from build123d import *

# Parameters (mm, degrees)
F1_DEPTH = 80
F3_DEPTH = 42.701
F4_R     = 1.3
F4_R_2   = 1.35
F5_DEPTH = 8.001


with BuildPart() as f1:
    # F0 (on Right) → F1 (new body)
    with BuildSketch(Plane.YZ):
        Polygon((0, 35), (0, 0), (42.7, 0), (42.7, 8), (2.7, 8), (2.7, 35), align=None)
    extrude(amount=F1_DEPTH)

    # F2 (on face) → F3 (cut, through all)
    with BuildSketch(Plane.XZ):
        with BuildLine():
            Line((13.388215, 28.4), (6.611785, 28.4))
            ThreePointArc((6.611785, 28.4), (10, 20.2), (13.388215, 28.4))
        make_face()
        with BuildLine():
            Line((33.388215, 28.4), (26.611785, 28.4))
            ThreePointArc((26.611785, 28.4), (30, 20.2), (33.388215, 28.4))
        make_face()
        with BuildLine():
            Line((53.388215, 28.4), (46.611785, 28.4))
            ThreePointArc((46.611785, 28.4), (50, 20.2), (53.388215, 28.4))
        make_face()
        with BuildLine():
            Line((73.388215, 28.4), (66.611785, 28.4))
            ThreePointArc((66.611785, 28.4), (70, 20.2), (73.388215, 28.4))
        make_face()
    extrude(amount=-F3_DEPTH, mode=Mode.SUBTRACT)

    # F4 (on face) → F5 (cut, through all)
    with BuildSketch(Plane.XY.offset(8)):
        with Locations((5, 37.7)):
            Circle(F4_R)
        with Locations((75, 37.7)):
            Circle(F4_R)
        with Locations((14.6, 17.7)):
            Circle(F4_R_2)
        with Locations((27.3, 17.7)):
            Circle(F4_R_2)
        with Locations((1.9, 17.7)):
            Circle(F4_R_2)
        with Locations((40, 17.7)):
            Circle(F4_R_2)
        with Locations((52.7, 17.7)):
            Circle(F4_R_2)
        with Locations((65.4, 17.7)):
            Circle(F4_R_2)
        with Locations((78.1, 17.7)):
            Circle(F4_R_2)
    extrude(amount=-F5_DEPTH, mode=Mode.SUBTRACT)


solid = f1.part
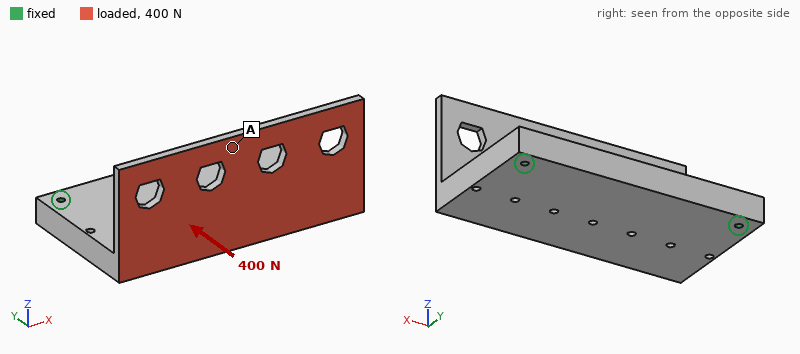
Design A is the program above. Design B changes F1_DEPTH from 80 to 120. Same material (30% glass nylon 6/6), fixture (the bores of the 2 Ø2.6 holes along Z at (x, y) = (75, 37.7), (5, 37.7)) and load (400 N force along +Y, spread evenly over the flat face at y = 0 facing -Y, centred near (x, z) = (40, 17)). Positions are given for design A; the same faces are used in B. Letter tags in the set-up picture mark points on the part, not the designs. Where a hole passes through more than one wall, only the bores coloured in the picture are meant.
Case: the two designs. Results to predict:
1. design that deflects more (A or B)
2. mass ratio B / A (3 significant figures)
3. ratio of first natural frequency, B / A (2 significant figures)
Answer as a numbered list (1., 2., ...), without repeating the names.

1. A
2. 1.52
3. 0.86
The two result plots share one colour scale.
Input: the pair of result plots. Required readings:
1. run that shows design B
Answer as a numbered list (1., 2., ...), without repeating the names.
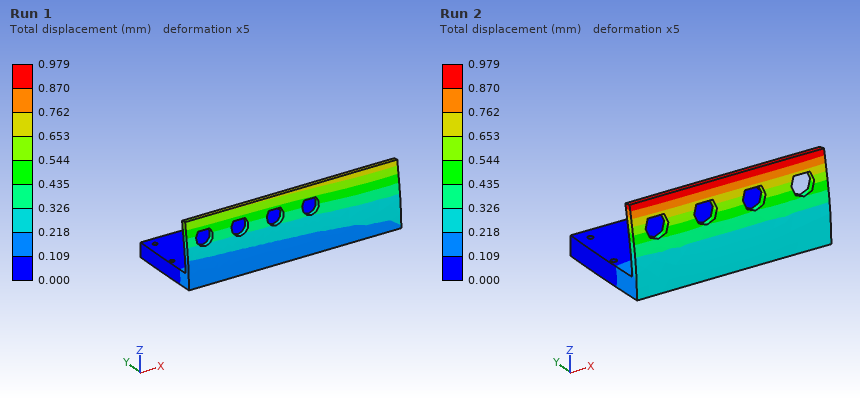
1. Run 1
